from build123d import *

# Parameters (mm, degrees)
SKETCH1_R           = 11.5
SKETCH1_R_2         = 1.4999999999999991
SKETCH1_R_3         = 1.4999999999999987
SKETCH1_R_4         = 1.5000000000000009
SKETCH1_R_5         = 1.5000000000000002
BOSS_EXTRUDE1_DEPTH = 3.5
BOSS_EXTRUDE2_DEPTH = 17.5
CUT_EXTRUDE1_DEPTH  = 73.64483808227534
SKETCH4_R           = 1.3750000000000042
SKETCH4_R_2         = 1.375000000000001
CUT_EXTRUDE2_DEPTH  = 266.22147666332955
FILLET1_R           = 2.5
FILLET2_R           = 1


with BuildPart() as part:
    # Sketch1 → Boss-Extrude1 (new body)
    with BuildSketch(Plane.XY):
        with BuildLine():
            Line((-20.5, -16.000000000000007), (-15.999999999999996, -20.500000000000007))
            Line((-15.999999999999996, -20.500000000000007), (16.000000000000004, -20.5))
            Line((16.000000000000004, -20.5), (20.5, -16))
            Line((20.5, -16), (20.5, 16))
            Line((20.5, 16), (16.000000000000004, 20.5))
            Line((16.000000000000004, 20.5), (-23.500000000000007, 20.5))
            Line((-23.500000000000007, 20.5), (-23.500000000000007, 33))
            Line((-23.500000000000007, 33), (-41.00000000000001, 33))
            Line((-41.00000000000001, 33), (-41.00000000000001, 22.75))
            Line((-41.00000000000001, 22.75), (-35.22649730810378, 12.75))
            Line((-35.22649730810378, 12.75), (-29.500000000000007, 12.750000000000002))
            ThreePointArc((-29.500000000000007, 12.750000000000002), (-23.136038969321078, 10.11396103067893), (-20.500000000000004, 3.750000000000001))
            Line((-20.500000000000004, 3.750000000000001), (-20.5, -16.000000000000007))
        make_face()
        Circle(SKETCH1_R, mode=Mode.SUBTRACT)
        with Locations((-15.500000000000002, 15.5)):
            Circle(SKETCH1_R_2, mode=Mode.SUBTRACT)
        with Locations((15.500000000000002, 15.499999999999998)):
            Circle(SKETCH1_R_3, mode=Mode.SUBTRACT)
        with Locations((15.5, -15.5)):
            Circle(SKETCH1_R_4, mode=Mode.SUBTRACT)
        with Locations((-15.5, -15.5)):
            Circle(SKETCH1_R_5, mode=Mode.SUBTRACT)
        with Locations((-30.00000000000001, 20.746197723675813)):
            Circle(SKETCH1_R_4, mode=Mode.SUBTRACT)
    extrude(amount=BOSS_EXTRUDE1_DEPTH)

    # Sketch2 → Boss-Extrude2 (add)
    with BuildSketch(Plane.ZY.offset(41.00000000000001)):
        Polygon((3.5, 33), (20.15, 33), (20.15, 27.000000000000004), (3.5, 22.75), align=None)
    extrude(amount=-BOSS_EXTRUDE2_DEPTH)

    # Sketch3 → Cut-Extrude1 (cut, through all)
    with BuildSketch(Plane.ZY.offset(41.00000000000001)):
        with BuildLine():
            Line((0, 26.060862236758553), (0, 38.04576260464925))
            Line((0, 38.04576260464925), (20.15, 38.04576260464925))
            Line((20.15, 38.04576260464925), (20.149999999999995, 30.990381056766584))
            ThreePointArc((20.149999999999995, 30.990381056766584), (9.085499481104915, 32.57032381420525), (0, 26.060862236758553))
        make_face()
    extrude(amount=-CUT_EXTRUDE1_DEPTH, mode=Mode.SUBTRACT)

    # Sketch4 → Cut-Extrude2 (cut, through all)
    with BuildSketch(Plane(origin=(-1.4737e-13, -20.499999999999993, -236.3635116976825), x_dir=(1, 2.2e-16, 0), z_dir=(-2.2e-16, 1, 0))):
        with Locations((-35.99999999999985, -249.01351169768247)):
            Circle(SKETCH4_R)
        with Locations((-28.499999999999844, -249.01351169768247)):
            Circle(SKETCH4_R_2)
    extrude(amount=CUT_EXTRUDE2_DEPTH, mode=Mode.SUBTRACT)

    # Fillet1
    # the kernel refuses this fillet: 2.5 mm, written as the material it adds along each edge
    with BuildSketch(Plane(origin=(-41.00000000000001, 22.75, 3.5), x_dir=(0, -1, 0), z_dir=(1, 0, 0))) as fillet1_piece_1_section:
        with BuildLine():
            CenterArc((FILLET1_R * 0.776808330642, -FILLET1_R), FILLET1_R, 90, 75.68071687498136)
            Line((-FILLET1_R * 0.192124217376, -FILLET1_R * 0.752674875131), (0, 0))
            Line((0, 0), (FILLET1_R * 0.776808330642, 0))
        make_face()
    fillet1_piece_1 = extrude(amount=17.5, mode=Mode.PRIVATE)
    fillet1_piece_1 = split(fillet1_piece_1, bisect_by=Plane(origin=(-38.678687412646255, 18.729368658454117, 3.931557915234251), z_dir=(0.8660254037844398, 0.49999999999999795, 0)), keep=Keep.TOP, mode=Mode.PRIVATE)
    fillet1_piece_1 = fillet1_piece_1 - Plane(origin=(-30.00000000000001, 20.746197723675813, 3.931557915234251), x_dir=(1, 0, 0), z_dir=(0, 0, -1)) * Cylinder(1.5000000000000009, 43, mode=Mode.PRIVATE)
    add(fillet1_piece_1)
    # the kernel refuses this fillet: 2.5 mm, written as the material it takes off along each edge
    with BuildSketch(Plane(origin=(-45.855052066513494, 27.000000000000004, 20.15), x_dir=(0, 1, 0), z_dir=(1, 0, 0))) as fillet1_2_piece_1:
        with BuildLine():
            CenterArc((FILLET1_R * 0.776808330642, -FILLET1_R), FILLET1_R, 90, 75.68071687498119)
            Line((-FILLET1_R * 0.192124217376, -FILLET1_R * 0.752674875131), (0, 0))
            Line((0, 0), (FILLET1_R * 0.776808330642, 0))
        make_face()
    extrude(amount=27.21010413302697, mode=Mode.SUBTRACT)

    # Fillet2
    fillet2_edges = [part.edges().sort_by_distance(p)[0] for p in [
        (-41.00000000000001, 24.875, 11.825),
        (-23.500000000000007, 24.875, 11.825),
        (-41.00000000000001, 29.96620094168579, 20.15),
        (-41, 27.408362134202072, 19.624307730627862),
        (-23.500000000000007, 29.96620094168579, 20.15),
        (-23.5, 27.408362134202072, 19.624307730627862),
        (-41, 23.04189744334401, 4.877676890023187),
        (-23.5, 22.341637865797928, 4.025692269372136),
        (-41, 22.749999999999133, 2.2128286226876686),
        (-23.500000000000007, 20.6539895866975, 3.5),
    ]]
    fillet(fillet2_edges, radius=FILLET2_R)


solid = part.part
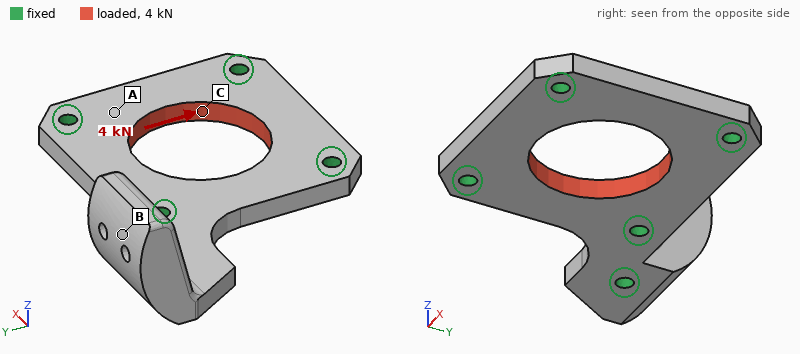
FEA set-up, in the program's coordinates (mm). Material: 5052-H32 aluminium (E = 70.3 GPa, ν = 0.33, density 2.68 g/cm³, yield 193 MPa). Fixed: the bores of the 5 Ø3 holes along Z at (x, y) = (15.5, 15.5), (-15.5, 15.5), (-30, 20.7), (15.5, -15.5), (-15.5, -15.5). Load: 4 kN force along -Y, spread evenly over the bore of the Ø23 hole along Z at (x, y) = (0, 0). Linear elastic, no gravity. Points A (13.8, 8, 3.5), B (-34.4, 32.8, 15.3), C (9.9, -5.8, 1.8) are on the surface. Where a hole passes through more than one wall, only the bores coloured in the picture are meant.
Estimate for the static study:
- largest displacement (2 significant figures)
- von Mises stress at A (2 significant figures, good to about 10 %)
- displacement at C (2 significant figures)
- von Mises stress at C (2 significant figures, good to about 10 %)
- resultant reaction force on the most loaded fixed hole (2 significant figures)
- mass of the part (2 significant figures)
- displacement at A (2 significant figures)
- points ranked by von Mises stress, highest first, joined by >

12 µm
25 MPa
5.7 µm
41 MPa
1.0 kN
19 g
3.4 µm
C > A > B
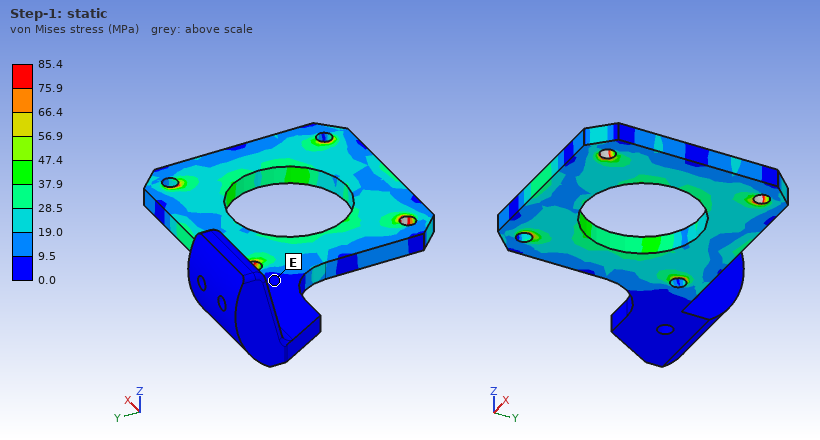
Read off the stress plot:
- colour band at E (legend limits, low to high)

0.0 to 9.5 MPa
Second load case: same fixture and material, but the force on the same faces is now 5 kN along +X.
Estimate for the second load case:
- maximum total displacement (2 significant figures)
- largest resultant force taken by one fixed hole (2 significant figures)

15 µm
1.3 kN
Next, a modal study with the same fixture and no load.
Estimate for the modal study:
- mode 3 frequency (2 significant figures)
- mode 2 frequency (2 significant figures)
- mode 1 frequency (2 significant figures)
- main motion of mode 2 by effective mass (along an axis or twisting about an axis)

17 kHz
7800 Hz
6000 Hz
along X
